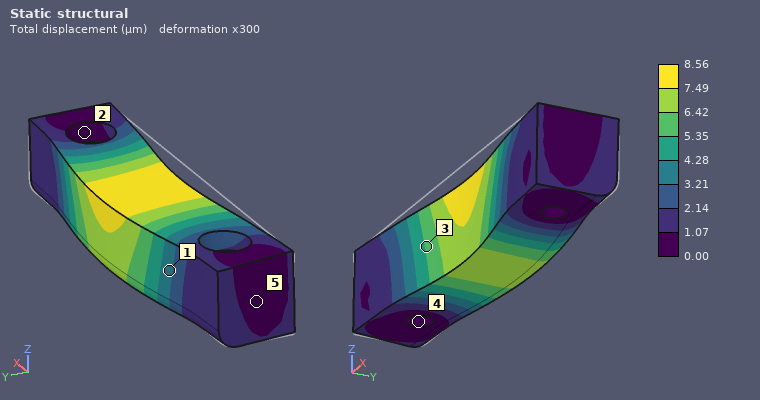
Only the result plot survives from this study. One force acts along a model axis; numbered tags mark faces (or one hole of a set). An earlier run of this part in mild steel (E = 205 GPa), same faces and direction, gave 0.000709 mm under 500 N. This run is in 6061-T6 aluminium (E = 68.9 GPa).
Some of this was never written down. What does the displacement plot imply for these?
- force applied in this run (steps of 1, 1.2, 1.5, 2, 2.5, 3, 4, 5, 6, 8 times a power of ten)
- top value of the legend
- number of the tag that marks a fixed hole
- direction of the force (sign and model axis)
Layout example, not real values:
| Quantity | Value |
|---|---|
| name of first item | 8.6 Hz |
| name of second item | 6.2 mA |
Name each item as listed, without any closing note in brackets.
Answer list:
| Quantity | Value |
|---|---|
| force applied in this run | 2 kN |
| top value of the legend | 8.56 µm |
| number of the tag that marks a fixed hole | 4 |
| direction of the force | +Y |
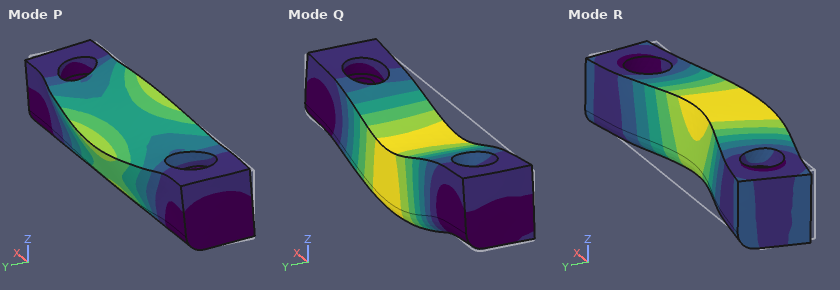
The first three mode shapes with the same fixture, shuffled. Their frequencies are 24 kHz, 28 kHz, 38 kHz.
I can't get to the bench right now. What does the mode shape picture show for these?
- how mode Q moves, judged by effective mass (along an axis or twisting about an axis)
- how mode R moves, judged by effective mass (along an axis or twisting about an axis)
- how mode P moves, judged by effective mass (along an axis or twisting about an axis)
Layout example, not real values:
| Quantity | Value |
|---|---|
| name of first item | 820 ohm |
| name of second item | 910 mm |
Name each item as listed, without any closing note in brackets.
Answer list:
| Quantity | Value |
|---|---|
| how mode Q moves, judged by effective mass | along Z |
| how mode R moves, judged by effective mass | along Y |
| how mode P moves, judged by effective mass | twisting about X |
